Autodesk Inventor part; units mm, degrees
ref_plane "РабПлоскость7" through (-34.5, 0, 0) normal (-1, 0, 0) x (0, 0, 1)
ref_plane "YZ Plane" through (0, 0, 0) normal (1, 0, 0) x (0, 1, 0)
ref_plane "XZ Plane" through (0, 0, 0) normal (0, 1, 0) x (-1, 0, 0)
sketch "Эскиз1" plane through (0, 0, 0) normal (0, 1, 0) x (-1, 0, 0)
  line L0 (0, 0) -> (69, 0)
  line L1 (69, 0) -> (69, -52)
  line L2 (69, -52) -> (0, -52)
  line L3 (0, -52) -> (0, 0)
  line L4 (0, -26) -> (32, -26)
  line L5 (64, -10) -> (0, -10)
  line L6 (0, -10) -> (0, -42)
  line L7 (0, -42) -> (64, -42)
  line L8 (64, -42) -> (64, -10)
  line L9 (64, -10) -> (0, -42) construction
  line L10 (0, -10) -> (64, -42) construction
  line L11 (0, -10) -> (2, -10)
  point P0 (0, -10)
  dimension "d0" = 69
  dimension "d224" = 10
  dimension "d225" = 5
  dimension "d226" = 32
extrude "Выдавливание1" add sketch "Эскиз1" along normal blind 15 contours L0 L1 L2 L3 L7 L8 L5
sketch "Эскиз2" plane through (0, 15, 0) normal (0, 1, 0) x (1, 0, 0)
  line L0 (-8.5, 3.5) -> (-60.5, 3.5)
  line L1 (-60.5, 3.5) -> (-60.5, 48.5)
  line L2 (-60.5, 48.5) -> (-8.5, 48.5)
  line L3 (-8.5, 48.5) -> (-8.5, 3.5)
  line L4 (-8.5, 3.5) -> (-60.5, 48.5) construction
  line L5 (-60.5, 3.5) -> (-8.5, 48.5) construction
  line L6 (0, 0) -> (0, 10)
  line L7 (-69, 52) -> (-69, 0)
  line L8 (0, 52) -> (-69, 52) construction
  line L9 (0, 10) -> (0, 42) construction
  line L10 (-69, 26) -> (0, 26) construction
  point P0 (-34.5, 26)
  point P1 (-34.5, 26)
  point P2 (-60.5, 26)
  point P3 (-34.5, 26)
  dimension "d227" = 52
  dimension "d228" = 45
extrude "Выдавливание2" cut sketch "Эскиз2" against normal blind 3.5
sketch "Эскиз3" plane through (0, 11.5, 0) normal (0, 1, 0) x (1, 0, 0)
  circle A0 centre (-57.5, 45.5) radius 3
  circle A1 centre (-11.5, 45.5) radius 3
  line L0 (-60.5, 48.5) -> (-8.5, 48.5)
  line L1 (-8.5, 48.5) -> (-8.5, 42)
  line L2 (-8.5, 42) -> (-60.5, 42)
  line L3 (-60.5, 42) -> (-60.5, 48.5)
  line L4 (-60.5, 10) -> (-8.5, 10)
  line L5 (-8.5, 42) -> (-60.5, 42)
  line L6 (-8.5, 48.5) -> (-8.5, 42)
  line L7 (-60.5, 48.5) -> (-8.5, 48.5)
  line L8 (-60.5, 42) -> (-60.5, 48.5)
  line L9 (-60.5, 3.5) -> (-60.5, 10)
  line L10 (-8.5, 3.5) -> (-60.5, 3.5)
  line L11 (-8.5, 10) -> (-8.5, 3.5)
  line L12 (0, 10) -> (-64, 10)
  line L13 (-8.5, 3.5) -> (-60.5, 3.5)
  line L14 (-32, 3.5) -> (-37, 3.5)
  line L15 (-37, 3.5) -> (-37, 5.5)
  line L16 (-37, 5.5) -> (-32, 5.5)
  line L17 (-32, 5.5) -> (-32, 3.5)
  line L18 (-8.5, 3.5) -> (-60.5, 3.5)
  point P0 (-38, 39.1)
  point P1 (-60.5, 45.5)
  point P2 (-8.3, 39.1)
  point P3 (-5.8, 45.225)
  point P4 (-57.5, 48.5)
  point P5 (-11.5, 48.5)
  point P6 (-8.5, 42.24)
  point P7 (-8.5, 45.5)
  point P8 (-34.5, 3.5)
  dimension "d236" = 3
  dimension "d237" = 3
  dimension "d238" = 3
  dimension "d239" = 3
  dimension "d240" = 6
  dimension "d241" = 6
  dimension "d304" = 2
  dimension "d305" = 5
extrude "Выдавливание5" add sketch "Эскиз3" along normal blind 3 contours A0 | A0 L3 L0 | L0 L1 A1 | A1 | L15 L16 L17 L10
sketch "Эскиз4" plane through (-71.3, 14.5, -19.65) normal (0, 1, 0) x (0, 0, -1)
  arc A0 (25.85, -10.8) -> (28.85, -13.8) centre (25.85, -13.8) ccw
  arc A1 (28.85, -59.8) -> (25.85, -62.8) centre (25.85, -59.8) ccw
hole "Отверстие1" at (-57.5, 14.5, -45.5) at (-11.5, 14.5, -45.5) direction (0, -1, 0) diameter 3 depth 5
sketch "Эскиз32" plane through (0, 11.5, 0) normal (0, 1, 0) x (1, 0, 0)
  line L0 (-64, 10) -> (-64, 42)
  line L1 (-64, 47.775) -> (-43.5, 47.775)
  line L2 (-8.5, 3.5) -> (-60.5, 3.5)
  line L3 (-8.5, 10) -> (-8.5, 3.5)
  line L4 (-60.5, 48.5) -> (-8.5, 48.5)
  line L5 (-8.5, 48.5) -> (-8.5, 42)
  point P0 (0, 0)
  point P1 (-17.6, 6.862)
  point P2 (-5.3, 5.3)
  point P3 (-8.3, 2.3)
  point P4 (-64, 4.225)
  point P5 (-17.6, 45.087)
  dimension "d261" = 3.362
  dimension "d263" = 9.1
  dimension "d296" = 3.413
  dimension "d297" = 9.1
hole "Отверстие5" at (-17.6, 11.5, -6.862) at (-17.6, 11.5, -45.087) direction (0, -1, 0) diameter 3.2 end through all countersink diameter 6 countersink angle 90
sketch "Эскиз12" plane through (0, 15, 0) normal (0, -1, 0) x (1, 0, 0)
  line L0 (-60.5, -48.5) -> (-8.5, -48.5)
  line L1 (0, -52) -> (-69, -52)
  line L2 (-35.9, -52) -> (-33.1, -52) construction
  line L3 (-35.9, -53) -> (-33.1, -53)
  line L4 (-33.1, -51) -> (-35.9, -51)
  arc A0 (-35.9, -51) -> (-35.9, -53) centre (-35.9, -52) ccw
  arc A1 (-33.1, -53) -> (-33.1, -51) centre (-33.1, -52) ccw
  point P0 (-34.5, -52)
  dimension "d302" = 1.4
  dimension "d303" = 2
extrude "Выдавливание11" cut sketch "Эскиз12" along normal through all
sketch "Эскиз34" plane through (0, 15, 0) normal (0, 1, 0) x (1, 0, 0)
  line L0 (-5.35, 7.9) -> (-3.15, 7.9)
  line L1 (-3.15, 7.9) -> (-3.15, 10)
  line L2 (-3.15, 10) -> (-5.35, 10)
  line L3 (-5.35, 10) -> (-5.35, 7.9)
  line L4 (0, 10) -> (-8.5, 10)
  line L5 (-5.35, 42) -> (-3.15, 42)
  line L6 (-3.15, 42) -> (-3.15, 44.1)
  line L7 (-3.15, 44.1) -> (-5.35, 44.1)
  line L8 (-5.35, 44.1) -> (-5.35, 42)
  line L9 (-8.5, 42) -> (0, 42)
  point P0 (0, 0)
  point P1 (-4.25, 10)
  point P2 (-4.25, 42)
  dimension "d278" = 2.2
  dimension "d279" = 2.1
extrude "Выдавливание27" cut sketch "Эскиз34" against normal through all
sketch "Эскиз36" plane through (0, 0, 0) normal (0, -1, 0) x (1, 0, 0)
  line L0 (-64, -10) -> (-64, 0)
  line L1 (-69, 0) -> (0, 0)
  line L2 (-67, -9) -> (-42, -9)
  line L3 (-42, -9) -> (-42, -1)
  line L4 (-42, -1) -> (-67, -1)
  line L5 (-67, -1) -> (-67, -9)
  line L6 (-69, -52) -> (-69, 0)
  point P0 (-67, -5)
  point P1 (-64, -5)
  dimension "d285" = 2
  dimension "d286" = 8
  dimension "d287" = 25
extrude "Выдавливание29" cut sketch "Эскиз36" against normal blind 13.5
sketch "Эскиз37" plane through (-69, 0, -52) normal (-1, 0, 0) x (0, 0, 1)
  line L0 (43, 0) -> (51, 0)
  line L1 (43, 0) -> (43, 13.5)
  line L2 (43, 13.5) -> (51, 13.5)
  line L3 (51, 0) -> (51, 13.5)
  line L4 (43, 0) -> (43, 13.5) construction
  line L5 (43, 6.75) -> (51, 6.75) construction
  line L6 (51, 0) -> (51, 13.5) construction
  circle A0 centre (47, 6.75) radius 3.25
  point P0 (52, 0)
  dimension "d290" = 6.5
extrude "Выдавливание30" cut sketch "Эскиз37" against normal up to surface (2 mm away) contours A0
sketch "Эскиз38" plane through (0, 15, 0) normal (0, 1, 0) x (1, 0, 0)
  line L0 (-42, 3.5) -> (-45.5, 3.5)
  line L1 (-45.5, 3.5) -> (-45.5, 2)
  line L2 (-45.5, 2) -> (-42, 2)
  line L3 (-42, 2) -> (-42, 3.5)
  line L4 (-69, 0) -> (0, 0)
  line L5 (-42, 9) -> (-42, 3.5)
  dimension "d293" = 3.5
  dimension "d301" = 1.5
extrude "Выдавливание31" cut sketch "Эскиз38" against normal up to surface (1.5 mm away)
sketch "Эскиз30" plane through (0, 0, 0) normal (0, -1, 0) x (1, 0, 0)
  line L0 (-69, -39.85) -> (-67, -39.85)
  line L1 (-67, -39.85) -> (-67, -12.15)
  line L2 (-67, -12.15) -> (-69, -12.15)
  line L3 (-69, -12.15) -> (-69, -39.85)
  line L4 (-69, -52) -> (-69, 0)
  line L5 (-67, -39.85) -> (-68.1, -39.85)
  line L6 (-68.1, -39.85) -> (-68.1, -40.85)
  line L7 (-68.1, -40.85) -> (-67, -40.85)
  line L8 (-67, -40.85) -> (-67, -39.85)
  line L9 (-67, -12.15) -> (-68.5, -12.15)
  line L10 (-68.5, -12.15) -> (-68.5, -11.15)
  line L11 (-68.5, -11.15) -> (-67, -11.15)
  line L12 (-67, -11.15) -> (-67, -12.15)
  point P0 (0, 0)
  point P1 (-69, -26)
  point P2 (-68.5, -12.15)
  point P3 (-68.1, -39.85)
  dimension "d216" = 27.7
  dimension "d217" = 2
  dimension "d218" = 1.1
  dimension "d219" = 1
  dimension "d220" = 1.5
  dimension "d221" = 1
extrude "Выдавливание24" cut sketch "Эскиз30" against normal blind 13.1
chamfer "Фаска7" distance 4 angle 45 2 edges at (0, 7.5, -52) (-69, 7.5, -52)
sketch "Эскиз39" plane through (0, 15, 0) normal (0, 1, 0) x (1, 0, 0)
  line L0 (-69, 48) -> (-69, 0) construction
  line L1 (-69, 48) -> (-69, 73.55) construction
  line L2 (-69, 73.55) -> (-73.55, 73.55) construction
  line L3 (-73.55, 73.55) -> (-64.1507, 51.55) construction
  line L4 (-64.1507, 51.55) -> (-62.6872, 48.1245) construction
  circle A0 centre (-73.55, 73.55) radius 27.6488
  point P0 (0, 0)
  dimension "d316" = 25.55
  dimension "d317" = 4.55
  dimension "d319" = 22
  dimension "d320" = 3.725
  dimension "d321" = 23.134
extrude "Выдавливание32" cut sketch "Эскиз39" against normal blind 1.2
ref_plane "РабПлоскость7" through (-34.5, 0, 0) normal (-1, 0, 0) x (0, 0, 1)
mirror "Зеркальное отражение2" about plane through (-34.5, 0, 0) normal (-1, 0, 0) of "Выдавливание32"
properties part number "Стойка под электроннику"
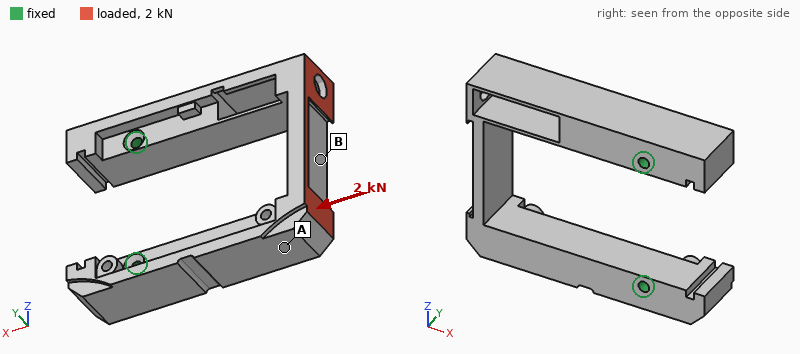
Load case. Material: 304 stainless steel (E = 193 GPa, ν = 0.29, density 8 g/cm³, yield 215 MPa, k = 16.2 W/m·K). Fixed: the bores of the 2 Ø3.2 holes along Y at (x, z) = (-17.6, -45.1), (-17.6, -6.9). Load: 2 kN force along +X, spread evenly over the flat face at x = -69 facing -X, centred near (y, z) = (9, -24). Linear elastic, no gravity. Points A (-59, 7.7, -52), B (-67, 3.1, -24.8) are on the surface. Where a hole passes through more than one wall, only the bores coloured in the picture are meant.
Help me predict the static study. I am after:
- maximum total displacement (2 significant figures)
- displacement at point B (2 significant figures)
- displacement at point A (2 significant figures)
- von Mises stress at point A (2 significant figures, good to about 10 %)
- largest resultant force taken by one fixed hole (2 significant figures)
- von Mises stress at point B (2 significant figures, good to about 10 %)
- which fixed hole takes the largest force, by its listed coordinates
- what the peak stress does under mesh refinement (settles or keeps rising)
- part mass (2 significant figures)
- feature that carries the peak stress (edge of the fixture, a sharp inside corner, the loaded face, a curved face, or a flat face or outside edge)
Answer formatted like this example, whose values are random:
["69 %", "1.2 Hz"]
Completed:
["36 µm", "25 µm", "14 µm", "11 MPa", "1.1 kN", "27 MPa", "(-17.6, -6.9)", "keeps rising", "130 g", "a sharp inside corner"]
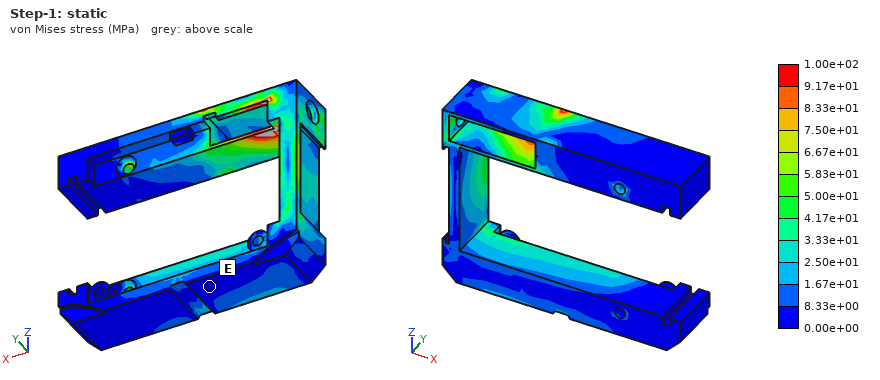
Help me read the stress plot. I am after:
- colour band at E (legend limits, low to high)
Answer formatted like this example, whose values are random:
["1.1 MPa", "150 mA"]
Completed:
["0.00e+00 to 8.33e+00 MPa"]
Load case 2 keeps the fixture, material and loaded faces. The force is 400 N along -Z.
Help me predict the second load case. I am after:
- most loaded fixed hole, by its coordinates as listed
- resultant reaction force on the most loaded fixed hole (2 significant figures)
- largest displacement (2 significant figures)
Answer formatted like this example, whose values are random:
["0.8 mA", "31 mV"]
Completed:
["(-17.6, -45.1)", "340 N", "76 µm"]
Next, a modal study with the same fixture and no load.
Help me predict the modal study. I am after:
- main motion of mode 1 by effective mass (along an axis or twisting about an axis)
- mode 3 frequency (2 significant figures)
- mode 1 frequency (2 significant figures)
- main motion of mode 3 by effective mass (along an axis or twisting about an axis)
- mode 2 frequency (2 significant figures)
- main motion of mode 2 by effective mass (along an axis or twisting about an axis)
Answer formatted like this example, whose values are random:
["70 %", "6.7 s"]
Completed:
["along Z", "4600 Hz", "2000 Hz", "twisting about X", "2900 Hz", "along Y"]
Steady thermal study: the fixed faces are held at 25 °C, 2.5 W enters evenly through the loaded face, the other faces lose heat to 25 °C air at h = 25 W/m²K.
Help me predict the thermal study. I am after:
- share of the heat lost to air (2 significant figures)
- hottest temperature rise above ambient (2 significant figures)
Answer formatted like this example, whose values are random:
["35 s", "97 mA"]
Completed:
["71 %", "27 K"]
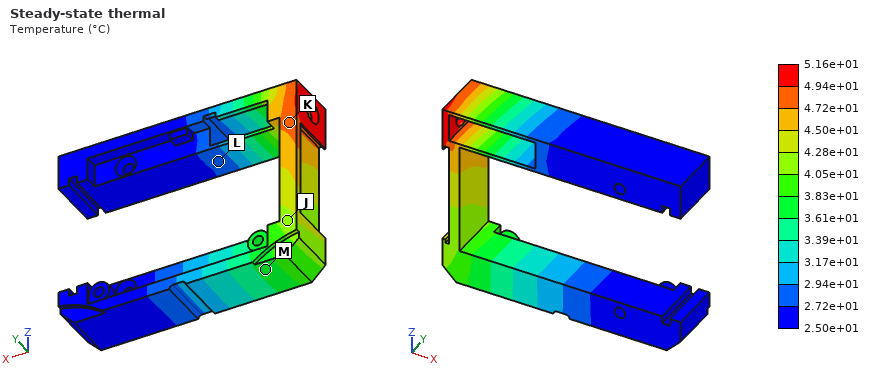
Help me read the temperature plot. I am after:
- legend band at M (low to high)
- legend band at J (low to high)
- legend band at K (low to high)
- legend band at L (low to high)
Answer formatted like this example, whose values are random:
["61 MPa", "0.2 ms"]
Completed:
["3.61e+01 to 3.83e+01 °C", "4.05e+01 to 4.28e+01 °C", "4.72e+01 to 4.94e+01 °C", "2.72e+01 to 2.94e+01 °C"]
